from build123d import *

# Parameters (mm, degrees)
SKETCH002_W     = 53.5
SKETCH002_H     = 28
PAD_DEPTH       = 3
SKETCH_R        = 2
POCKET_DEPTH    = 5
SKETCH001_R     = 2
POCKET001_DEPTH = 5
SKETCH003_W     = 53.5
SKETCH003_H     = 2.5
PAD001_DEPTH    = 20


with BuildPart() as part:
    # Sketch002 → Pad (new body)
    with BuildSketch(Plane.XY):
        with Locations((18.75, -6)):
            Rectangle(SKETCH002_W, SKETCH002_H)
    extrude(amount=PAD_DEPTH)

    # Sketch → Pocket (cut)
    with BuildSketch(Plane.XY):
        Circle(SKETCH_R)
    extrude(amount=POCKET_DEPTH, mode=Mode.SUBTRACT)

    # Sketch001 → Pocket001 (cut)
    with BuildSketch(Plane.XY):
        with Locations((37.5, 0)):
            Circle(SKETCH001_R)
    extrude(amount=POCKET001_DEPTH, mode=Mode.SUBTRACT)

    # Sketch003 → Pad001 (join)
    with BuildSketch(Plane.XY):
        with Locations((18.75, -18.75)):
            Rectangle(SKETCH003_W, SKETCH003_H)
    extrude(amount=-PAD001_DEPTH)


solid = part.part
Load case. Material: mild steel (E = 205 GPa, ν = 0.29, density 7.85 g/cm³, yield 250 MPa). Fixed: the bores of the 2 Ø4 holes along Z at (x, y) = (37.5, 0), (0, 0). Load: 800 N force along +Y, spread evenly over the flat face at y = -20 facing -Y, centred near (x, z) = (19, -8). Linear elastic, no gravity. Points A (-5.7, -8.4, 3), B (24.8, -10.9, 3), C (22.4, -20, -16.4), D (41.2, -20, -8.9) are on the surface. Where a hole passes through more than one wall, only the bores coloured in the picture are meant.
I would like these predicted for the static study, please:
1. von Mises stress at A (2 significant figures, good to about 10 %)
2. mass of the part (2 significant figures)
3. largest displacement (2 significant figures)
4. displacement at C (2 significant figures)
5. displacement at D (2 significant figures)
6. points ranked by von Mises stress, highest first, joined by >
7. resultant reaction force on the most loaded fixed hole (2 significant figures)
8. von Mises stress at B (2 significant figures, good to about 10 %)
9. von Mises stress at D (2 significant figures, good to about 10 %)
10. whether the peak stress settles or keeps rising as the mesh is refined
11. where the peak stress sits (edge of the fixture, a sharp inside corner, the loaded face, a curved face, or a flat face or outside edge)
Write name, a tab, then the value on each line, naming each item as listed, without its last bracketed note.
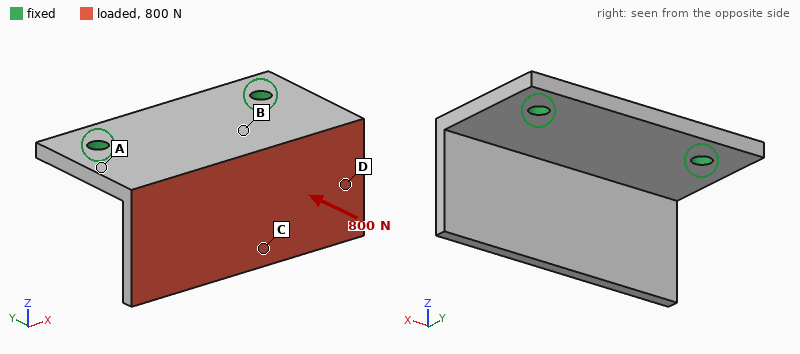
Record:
von Mises stress at A	110 MPa
mass of the part	56 g
largest displacement	0.20 mm
displacement at C	0.17 mm
displacement at D	0.11 mm
points ranked by von Mises stress, highest first, joined by >	A > B > D > C
resultant reaction force on the most loaded fixed hole	410 N
von Mises stress at B	80 MPa
von Mises stress at D	37 MPa
whether the peak stress settles or keeps rising as the mesh is refined	keeps rising
where the peak stress sits	edge of the fixture
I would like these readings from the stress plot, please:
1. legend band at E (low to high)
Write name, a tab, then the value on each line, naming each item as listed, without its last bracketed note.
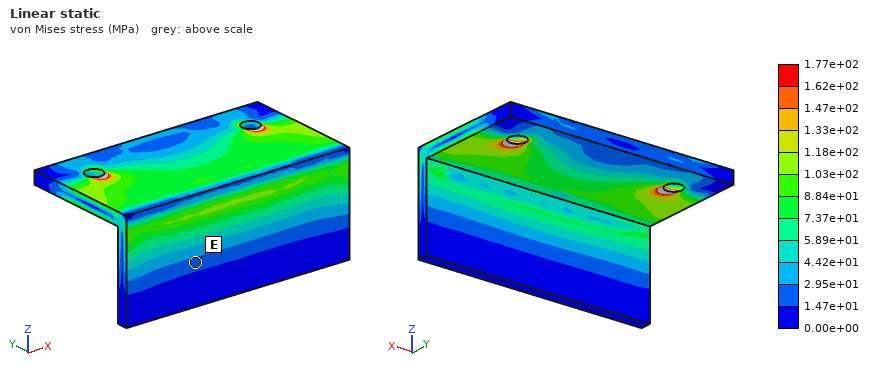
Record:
legend band at E	1.47e+01 to 2.95e+01 MPa
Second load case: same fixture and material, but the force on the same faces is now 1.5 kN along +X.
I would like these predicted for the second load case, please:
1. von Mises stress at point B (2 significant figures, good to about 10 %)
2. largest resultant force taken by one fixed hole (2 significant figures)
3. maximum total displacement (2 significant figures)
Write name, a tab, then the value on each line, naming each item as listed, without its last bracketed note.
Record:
von Mises stress at point B	37 MPa
largest resultant force taken by one fixed hole	1.1 kN
maximum total displacement	85 µm
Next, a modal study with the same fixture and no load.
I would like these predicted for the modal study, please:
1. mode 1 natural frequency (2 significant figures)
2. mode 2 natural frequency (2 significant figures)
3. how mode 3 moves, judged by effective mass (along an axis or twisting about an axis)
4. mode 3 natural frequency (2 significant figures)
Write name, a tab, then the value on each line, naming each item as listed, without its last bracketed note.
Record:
mode 1 natural frequency	2100 Hz
mode 2 natural frequency	3600 Hz
how mode 3 moves, judged by effective mass	along Z
mode 3 natural frequency	5100 Hz
